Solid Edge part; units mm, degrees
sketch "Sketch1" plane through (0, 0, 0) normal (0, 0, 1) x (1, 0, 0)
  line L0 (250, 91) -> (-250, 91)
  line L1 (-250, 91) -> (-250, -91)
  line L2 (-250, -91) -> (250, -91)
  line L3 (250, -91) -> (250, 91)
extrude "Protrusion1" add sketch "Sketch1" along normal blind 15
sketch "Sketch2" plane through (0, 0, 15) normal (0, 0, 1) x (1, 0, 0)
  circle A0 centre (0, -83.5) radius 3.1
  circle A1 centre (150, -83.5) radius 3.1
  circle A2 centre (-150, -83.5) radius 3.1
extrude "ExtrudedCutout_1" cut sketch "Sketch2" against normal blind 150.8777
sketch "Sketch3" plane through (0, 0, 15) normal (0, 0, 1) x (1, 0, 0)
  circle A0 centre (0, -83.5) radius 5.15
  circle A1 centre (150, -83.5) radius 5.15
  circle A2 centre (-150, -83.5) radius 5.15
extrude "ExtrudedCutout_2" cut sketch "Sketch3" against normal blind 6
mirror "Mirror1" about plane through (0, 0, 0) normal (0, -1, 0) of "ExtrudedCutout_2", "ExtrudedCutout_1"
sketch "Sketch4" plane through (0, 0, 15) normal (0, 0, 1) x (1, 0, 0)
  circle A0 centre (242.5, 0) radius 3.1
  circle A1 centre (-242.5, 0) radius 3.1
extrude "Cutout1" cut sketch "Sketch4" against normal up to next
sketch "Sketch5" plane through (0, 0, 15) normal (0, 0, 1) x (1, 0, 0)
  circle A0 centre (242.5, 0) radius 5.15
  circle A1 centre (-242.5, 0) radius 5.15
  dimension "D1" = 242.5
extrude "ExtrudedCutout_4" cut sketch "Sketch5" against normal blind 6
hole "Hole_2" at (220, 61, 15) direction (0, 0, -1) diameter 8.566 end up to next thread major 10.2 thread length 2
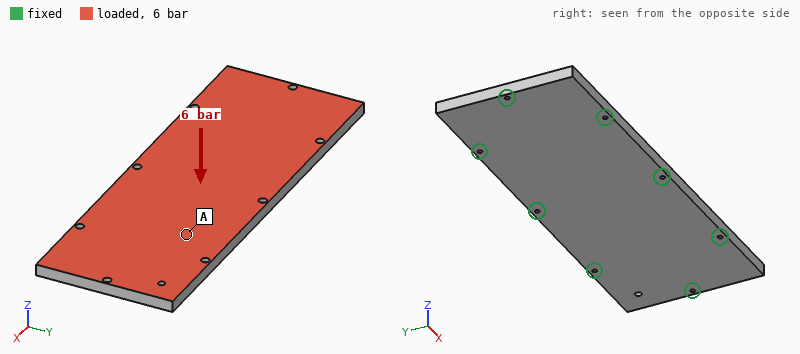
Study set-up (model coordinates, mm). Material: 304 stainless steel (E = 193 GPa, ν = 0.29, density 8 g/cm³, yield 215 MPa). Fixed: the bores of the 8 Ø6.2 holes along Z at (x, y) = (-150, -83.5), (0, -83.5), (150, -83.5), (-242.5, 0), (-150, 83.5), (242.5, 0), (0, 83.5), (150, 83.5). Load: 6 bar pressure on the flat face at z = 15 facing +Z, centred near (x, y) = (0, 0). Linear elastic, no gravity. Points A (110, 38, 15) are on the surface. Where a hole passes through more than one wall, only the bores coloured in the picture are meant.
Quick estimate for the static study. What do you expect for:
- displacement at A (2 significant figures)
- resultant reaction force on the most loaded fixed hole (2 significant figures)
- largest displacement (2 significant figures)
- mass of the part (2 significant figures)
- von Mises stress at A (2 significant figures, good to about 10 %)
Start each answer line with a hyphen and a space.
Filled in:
- 57 µm
- 10 kN
- 78 µm
- 11 kg
- 21 MPa
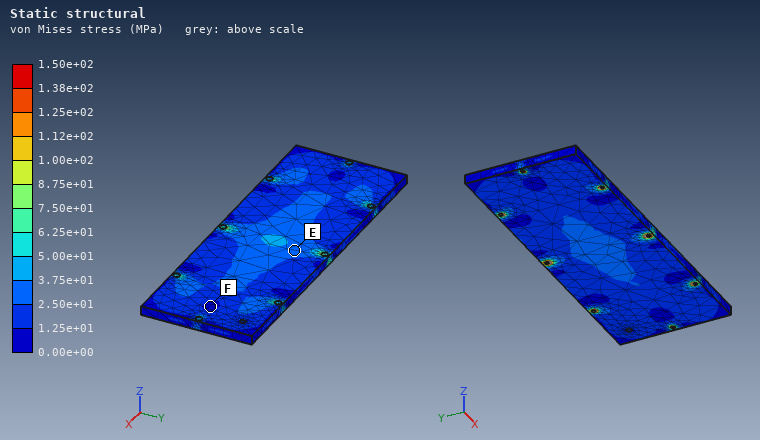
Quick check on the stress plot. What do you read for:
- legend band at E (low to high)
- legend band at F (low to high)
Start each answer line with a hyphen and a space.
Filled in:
- 2.50e+01 to 3.75e+01 MPa
- 0.00e+00 to 1.25e+01 MPa
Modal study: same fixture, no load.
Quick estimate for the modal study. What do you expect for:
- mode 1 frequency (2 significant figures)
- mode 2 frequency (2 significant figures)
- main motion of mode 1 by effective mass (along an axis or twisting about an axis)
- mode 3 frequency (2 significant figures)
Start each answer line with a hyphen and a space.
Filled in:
- 1500 Hz
- 1600 Hz
- along Z
- 1900 Hz
